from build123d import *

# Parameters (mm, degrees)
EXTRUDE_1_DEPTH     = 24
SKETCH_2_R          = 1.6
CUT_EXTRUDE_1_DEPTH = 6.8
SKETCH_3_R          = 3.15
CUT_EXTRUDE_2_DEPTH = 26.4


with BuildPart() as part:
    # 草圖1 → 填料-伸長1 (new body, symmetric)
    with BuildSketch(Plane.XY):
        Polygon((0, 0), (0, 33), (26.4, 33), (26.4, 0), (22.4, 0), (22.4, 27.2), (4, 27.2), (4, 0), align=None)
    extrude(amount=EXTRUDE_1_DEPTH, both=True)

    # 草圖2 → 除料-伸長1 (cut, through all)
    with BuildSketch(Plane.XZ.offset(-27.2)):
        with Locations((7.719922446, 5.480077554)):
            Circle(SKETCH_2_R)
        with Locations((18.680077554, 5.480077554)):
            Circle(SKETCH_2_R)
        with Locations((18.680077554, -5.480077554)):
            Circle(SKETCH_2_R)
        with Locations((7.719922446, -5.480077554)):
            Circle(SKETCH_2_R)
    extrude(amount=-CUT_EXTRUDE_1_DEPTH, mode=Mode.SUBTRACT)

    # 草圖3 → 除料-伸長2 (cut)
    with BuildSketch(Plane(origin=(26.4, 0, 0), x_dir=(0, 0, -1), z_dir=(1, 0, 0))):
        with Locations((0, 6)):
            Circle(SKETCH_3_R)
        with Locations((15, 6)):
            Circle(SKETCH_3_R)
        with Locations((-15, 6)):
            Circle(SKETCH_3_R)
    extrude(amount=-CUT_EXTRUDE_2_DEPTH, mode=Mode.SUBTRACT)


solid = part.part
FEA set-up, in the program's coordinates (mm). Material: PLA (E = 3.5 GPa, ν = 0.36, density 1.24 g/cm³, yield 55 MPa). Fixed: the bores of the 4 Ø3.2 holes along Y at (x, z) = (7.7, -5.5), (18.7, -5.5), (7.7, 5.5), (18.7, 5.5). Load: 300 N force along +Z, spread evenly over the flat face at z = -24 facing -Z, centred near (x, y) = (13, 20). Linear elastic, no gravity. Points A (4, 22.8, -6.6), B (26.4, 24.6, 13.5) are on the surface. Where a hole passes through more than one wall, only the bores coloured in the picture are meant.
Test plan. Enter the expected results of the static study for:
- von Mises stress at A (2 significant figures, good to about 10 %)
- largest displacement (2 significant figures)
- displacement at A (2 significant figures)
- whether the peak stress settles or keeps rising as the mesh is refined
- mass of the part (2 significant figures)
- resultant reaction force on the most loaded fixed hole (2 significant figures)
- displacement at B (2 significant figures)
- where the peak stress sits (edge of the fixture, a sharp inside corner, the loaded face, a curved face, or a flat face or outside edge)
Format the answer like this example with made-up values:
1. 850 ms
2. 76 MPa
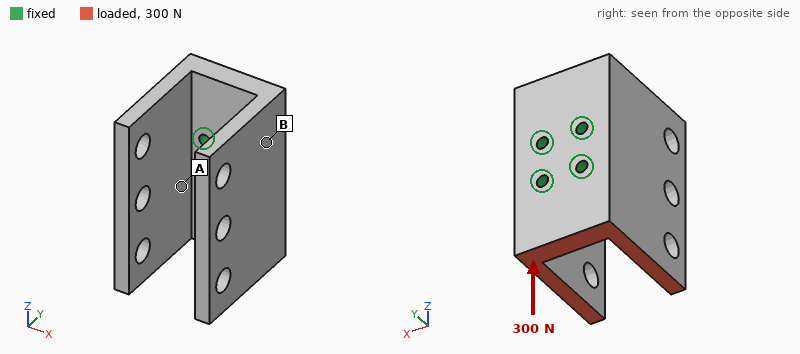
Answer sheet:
1. 2.1 MPa
2. 80 µm
3. 19 µm
4. keeps rising
5. 21 g
6. 130 N
7. 24 µm
8. edge of the fixture
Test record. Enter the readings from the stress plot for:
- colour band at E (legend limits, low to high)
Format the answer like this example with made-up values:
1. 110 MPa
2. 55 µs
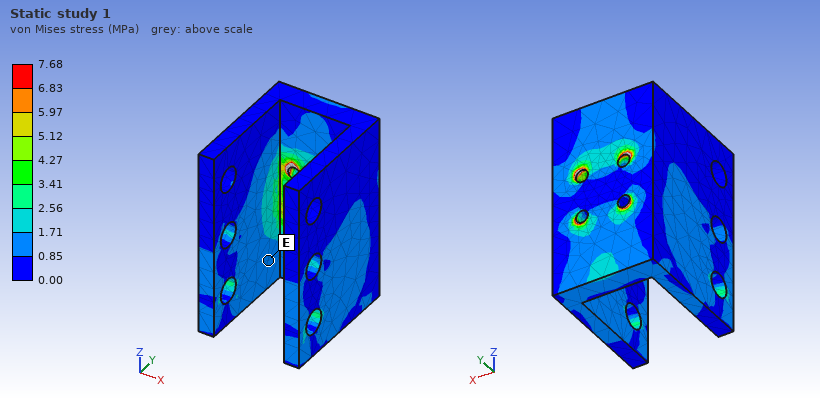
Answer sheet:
1. 0.85 to 1.71 MPa
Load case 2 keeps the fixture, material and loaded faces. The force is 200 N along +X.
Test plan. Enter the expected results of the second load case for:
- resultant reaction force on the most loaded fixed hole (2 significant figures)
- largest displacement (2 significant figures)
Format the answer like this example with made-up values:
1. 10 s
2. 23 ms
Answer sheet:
1. 210 N
2. 0.62 mm
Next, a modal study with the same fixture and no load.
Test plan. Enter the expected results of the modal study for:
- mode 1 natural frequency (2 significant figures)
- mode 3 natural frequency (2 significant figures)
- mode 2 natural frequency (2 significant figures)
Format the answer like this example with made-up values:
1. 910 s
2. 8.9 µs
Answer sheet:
1. 1200 Hz
2. 1800 Hz
3. 1300 Hz
